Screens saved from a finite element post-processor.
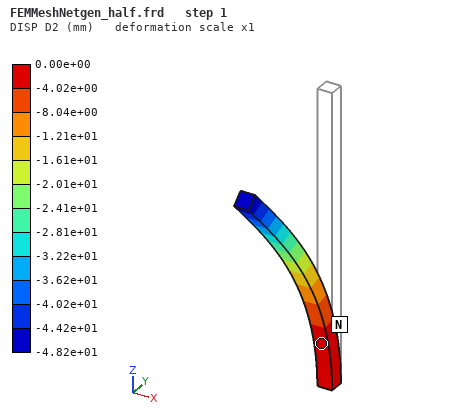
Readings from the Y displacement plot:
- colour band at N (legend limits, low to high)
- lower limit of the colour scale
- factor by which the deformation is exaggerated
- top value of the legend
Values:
-4.02e+00 to 0.00e+00 mm
-4.82e+01 mm
1
0.00e+00 mm
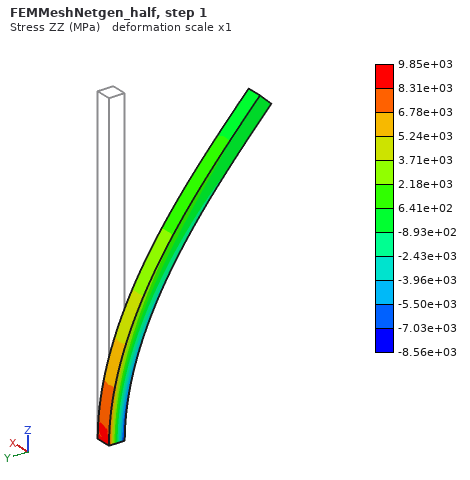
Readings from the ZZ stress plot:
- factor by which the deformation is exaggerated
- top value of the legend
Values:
1
9.85e+03 MPa
